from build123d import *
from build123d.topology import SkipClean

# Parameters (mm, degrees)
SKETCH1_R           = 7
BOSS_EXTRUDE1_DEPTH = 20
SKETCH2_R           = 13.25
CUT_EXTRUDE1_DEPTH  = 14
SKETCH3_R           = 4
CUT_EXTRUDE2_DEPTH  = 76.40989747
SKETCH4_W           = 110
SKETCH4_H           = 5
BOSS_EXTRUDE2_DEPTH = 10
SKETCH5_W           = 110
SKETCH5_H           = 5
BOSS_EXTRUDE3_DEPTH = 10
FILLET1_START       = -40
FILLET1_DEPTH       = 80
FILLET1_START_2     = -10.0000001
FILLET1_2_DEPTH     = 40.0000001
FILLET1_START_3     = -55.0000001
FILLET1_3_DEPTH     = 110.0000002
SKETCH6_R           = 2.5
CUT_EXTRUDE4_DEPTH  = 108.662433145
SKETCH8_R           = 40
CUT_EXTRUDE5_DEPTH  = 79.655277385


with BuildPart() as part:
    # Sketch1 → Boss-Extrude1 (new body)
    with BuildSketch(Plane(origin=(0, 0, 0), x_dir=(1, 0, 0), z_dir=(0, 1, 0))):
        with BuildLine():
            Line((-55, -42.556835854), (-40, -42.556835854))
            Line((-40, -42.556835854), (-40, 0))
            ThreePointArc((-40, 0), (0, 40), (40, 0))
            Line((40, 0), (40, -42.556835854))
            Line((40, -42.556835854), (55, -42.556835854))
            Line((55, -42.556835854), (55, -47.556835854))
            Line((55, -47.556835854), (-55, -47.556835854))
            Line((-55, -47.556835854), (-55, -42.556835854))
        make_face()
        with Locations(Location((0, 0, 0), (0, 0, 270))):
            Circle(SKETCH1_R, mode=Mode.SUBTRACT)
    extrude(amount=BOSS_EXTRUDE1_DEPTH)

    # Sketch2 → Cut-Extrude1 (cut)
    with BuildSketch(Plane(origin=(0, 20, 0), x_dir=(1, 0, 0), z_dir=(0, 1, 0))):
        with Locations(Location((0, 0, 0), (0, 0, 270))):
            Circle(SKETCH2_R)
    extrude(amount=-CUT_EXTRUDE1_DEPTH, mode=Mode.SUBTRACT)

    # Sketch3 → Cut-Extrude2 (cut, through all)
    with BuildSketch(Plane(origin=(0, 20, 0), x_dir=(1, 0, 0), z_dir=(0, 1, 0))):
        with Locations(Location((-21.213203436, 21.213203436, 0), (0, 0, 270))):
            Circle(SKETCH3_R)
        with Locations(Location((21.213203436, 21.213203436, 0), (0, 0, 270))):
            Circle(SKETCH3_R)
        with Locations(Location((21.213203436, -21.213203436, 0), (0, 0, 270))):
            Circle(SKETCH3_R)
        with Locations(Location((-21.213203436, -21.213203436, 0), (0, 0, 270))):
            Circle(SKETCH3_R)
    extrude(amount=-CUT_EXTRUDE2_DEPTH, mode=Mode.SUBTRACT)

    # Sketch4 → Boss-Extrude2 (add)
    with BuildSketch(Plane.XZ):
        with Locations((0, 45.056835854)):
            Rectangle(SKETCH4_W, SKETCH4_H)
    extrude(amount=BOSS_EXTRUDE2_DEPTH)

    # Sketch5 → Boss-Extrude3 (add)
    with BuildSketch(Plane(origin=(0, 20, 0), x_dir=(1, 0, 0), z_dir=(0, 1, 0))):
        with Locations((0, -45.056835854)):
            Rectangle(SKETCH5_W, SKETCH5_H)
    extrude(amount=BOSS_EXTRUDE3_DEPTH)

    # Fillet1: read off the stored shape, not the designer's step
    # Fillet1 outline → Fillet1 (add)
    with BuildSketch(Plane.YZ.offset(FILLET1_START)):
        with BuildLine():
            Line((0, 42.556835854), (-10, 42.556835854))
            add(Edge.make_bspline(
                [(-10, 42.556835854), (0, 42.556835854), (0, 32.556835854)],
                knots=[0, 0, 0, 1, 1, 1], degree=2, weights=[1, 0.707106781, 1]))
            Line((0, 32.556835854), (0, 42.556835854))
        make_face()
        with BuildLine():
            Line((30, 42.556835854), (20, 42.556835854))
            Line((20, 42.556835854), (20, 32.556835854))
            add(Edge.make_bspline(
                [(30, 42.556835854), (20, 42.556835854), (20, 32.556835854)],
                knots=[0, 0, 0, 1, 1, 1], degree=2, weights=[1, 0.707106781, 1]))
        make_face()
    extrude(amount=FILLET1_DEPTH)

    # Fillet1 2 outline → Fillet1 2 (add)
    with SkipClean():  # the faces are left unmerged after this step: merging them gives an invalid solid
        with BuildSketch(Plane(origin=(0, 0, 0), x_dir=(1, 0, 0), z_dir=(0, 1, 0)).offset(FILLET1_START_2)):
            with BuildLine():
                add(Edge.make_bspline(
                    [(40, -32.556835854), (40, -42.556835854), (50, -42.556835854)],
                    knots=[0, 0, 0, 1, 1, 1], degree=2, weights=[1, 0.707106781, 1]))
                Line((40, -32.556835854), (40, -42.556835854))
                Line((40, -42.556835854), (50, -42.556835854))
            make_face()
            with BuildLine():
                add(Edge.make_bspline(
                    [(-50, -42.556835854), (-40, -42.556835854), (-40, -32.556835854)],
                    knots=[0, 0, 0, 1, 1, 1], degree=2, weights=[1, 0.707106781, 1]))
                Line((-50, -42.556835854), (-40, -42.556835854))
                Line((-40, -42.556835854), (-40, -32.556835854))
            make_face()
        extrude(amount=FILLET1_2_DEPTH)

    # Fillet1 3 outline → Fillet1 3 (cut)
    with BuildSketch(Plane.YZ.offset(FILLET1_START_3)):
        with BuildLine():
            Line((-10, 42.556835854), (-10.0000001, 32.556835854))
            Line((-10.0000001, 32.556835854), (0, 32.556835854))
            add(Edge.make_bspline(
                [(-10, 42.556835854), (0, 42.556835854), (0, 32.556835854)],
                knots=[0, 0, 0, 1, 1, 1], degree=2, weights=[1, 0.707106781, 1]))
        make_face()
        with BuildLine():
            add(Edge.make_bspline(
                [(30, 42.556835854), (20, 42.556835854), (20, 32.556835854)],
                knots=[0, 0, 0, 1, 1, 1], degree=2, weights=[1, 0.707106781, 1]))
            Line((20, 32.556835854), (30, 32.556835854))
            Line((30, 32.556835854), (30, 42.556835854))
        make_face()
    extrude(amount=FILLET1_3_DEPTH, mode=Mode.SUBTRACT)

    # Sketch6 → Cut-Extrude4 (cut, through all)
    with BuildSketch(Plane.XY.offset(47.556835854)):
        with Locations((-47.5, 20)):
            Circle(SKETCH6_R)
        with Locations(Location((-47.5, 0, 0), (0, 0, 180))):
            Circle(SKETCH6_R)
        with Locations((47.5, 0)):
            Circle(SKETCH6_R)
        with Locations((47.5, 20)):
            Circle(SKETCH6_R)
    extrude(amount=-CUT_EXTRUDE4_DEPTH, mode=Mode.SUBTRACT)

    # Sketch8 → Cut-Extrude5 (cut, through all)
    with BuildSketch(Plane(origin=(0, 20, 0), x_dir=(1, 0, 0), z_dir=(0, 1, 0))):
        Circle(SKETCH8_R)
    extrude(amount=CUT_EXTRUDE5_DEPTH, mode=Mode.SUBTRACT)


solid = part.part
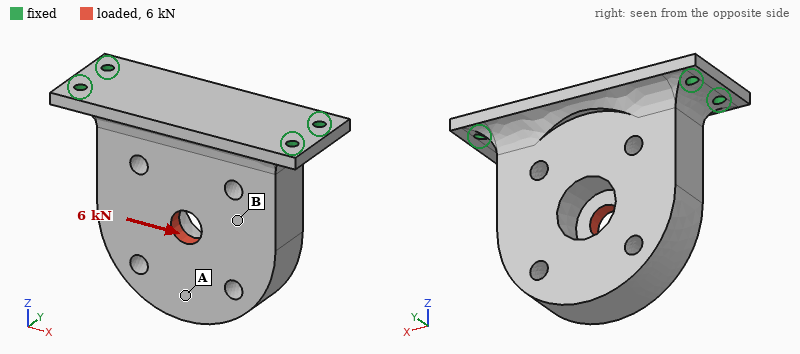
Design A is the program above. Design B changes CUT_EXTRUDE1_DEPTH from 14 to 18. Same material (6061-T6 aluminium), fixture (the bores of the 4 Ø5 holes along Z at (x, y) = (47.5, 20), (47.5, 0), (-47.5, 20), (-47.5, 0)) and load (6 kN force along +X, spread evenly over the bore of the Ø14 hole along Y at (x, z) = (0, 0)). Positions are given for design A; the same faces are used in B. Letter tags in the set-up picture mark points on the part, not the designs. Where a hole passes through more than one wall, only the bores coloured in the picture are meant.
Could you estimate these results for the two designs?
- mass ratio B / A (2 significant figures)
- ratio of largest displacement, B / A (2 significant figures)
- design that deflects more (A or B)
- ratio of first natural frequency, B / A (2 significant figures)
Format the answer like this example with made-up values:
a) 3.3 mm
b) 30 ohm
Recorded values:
a) 0.99
b) 1.1
c) B
d) 1.0
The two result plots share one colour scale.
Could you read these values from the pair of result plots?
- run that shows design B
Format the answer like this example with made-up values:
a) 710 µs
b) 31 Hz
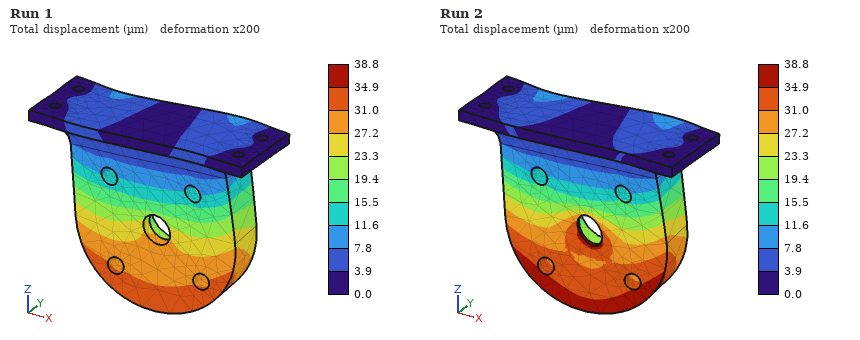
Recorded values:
a) Run 2
